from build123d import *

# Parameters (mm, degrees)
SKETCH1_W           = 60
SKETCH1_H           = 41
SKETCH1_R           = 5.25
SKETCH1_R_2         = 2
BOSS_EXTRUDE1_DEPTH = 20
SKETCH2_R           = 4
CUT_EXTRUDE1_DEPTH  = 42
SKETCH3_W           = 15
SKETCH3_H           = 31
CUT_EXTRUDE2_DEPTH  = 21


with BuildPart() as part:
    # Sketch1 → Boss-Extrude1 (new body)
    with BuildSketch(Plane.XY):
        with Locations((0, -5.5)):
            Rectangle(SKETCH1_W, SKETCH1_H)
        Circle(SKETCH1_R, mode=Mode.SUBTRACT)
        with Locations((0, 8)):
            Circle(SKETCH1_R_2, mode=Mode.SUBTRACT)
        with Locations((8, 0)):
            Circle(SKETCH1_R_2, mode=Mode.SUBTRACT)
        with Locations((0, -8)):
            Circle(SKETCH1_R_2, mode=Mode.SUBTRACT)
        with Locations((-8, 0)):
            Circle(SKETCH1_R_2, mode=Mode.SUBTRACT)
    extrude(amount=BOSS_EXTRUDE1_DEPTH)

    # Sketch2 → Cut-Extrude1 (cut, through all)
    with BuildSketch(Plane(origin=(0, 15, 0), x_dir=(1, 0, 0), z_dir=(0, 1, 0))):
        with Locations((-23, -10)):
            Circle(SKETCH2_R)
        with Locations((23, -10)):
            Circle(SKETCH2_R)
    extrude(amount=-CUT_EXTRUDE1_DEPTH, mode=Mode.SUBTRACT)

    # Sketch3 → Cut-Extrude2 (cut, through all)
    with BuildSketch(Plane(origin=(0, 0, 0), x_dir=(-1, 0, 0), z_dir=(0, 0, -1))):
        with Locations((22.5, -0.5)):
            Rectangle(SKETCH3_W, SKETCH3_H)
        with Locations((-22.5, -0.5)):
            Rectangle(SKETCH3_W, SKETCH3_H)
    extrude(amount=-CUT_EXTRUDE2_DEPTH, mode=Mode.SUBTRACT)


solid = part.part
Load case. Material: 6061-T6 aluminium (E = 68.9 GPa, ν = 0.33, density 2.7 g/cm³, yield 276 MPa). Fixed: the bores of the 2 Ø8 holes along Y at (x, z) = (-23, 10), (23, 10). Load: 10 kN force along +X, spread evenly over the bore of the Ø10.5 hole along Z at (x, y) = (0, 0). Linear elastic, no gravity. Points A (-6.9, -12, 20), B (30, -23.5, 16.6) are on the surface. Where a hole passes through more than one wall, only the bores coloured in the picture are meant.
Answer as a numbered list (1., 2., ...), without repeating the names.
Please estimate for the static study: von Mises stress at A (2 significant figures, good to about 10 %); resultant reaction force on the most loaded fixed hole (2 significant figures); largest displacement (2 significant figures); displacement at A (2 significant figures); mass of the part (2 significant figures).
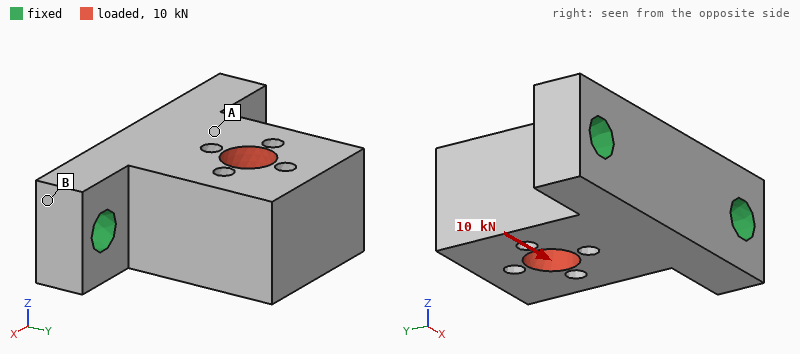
1. 28 MPa
2. 7.6 kN
3. 77 µm
4. 13 µm
5. 73 g
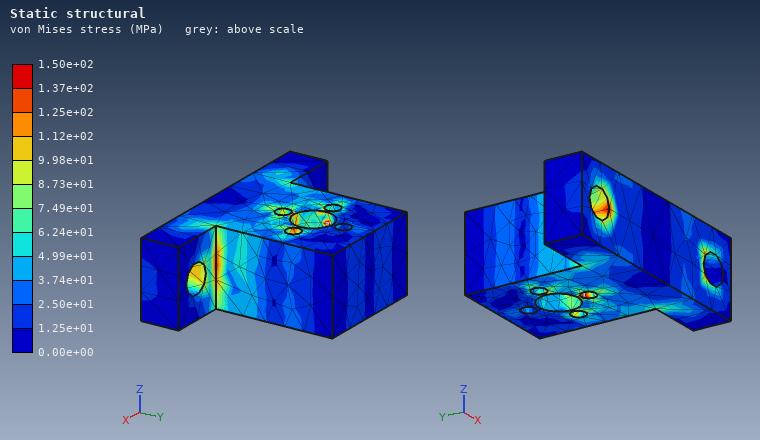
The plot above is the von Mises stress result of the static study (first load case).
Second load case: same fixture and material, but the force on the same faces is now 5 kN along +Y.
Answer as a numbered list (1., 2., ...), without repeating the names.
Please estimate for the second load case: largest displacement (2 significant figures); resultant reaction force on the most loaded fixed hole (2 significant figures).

1. 13 µm
2. 2.7 kN
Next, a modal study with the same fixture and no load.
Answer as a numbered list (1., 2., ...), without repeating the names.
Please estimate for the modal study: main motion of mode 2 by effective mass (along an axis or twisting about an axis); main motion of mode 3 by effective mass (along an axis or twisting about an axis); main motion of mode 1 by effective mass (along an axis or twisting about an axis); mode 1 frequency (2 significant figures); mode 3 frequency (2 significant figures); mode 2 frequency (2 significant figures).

1. along X
2. twisting about Y
3. along Z
4. 5100 Hz
5. 15 kHz
6. 10 kHz
